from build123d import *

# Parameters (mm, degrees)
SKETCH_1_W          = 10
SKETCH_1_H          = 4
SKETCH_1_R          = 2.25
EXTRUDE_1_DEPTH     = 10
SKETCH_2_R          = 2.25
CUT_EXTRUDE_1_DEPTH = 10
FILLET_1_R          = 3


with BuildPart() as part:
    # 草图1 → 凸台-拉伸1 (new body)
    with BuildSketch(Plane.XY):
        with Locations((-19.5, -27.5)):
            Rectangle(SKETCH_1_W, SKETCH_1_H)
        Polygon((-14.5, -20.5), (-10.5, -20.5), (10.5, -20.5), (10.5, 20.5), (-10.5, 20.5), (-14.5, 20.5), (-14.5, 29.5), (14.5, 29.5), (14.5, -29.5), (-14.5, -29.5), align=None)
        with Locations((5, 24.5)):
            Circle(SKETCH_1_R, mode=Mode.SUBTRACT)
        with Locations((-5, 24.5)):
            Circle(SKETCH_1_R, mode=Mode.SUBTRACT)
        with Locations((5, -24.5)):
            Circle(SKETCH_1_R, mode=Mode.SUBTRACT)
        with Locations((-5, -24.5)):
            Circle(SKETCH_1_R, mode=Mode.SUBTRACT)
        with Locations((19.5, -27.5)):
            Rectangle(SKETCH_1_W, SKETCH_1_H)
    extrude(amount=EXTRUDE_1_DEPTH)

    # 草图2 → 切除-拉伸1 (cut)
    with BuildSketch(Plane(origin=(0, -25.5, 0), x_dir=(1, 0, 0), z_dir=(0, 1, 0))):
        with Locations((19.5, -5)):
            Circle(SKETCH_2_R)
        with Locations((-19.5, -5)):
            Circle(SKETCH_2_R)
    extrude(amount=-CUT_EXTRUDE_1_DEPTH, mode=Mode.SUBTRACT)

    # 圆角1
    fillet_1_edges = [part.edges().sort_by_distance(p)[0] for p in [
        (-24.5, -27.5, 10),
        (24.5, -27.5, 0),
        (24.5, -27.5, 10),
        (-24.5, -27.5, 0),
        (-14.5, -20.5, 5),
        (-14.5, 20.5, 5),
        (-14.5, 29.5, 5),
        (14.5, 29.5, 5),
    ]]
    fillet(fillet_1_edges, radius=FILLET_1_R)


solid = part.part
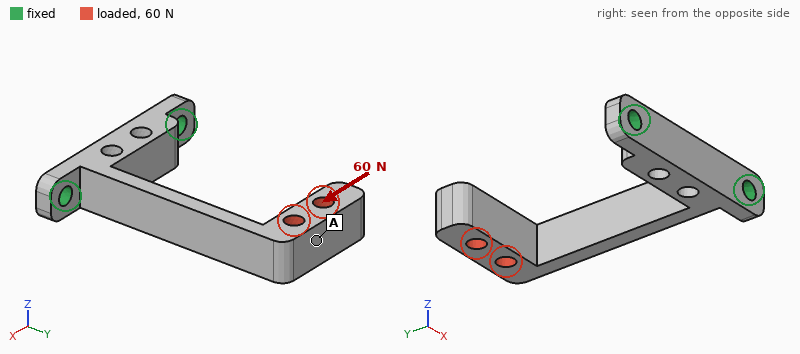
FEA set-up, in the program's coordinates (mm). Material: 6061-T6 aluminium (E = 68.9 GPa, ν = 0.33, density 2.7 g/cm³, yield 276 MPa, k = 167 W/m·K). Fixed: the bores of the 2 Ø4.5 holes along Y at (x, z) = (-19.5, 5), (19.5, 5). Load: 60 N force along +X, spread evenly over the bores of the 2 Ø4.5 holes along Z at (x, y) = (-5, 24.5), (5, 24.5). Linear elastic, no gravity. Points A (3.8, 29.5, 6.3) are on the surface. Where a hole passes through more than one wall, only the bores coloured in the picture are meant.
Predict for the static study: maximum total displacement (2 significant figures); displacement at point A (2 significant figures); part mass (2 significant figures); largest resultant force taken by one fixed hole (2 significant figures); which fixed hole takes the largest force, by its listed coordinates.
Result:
0.82 mm
0.70 mm
18 g
170 N
(-19.5, 5)
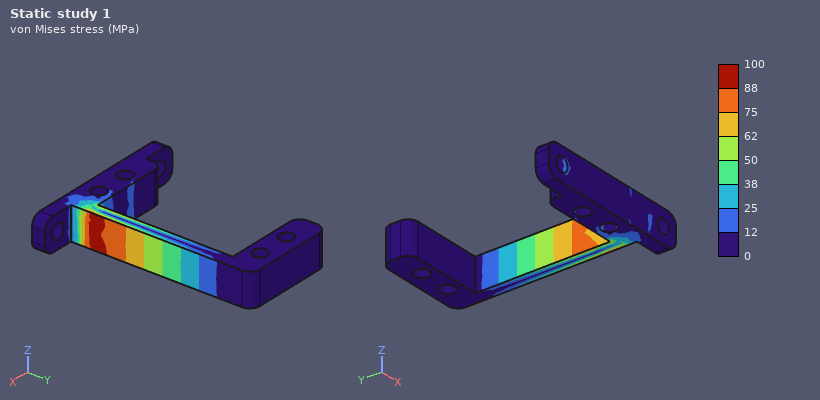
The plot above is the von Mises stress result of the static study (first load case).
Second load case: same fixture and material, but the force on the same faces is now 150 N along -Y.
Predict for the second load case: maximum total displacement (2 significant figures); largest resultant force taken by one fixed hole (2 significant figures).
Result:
0.91 mm
130 N
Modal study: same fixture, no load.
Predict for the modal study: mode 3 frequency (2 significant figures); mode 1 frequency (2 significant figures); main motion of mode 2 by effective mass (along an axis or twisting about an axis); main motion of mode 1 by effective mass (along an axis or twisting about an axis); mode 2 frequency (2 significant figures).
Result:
2300 Hz
550 Hz
along Z
along X
860 Hz
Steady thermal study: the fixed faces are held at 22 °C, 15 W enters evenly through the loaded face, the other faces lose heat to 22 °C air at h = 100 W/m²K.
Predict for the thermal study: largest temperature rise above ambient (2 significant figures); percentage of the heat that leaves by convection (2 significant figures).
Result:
60 K
65 %
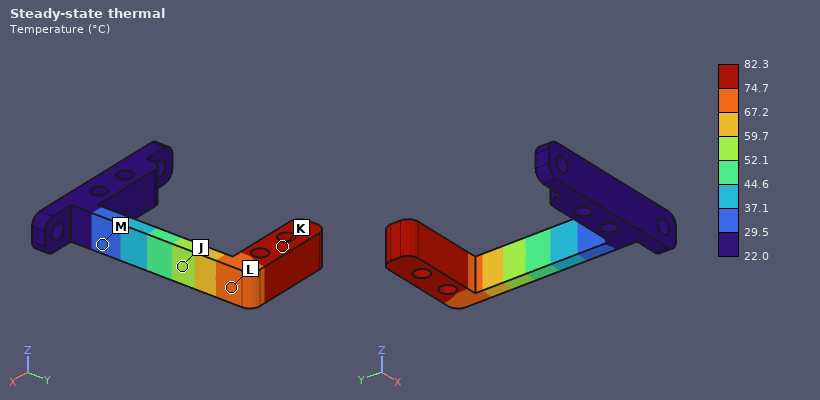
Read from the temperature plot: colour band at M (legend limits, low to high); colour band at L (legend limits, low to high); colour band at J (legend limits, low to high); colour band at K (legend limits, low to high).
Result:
29.5 to 37.1 °C
67.2 to 74.7 °C
52.1 to 59.7 °C
74.7 to 82.3 °C
